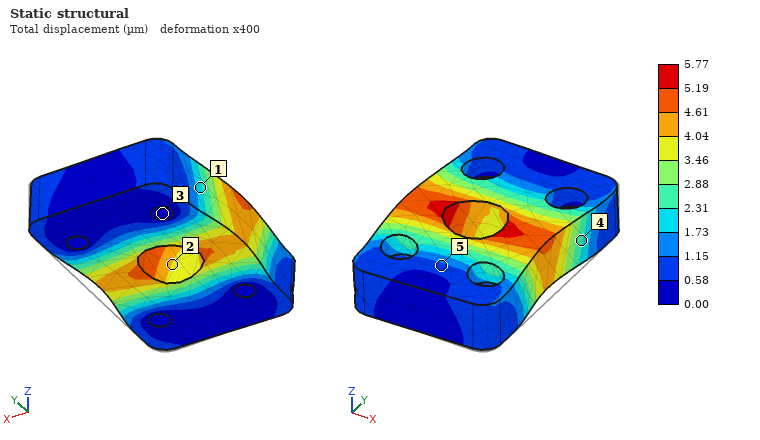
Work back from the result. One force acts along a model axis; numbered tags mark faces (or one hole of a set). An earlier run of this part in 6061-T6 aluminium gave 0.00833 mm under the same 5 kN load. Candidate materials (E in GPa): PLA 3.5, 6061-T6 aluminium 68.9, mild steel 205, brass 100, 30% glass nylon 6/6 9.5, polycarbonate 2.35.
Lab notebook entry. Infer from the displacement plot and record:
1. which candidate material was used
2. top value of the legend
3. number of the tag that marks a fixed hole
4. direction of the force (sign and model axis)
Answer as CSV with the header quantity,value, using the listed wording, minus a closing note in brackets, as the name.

quantity,value
which candidate material was used,brass
top value of the legend,5.77 µm
number of the tag that marks a fixed hole,3
direction of the force,-X
